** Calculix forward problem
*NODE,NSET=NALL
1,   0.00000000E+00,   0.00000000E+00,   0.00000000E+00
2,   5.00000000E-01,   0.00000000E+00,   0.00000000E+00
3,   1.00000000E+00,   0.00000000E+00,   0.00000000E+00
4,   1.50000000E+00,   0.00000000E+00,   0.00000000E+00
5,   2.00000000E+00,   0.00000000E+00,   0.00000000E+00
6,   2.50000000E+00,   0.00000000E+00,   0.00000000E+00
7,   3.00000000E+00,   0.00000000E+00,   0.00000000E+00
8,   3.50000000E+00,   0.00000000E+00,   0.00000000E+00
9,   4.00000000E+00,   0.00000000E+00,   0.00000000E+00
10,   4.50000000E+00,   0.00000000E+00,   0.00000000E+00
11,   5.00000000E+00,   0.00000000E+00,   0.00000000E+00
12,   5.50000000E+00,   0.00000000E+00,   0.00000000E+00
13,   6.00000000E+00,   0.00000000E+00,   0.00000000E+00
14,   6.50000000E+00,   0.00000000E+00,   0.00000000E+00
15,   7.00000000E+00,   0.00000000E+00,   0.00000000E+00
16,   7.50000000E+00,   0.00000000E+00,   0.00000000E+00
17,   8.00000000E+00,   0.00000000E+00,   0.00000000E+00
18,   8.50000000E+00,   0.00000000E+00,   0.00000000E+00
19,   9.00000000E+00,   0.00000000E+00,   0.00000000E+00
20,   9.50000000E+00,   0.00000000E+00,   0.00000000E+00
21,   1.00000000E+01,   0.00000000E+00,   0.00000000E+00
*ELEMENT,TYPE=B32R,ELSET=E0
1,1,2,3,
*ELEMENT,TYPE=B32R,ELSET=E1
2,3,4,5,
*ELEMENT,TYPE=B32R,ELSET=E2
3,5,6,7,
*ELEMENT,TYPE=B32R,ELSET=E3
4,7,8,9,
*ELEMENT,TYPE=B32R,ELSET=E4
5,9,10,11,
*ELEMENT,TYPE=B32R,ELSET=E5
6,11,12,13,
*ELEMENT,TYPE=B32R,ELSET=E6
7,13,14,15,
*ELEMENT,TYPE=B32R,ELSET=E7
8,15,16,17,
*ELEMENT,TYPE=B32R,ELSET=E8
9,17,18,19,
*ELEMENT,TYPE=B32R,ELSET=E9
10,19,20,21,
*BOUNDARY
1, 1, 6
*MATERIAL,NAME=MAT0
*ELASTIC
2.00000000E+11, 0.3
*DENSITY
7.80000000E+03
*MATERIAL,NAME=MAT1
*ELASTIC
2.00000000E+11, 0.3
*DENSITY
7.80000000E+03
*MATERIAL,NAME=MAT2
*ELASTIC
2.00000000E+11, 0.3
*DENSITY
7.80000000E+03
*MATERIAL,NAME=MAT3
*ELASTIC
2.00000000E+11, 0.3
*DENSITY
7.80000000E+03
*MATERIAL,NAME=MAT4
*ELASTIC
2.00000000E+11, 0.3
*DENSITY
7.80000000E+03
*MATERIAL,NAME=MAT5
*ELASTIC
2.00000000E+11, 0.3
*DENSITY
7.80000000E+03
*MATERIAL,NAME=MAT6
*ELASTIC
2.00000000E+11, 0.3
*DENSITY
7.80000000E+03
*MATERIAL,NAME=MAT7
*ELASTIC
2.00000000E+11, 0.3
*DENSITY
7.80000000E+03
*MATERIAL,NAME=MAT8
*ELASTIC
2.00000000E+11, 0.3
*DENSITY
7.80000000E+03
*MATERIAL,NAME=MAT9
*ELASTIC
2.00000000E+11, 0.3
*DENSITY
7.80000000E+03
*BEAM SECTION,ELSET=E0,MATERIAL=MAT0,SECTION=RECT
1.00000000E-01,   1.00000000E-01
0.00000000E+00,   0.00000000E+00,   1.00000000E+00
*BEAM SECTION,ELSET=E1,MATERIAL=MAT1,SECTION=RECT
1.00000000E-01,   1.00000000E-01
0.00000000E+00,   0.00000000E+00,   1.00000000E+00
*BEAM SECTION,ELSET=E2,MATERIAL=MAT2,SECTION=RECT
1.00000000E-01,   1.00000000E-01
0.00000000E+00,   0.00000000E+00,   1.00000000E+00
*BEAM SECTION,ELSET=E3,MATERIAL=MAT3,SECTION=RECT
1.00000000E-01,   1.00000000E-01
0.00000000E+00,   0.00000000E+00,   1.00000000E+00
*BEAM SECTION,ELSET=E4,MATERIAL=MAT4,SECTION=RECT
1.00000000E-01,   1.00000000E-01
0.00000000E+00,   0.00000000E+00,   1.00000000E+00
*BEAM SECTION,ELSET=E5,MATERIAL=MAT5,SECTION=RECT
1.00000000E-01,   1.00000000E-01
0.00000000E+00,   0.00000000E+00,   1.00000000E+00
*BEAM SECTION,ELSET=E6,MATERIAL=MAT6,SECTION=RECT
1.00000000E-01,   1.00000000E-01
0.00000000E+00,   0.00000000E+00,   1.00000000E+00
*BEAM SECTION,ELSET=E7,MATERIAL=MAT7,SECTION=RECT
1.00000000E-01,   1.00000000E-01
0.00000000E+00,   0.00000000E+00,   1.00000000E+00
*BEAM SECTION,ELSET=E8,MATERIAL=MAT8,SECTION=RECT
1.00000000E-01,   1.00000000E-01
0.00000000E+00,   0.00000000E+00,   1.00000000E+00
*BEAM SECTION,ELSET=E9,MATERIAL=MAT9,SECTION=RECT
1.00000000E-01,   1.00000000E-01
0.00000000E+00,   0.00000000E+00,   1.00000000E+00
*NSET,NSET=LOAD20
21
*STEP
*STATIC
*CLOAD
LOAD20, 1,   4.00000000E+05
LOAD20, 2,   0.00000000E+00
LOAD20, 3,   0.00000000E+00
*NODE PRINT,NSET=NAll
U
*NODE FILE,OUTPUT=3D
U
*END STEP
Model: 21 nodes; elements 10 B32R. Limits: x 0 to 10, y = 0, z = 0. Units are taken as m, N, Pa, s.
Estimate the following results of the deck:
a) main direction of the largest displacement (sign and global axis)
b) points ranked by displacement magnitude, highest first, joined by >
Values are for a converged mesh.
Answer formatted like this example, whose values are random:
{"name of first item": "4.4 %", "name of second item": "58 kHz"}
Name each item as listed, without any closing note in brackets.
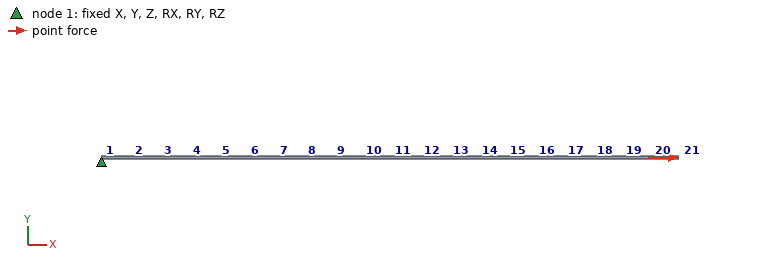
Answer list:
{"main direction of the largest displacement": "+X", "points ranked by displacement magnitude, highest first, joined by >": "node 20 > node 16 > node 13 > node 11 > node 8"}
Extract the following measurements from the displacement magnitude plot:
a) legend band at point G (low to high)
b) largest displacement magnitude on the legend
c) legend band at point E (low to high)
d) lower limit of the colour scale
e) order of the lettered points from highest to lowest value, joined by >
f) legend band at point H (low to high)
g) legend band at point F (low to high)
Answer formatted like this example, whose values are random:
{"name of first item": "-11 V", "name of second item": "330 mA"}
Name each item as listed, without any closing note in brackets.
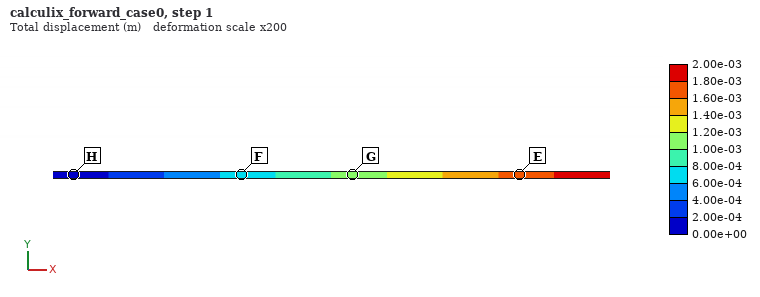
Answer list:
{"legend band at point G": "1.00e-03 to 1.20e-03 m", "largest displacement magnitude on the legend": "2.00e-03 m", "legend band at point E": "1.60e-03 to 1.80e-03 m", "lower limit of the colour scale": "0.00e+00 m", "order of the lettered points from highest to lowest value, joined by >": "E > G > F > H", "legend band at point H": "0.00e+00 to 2.00e-04 m", "legend band at point F": "6.00e-04 to 8.00e-04 m"}
